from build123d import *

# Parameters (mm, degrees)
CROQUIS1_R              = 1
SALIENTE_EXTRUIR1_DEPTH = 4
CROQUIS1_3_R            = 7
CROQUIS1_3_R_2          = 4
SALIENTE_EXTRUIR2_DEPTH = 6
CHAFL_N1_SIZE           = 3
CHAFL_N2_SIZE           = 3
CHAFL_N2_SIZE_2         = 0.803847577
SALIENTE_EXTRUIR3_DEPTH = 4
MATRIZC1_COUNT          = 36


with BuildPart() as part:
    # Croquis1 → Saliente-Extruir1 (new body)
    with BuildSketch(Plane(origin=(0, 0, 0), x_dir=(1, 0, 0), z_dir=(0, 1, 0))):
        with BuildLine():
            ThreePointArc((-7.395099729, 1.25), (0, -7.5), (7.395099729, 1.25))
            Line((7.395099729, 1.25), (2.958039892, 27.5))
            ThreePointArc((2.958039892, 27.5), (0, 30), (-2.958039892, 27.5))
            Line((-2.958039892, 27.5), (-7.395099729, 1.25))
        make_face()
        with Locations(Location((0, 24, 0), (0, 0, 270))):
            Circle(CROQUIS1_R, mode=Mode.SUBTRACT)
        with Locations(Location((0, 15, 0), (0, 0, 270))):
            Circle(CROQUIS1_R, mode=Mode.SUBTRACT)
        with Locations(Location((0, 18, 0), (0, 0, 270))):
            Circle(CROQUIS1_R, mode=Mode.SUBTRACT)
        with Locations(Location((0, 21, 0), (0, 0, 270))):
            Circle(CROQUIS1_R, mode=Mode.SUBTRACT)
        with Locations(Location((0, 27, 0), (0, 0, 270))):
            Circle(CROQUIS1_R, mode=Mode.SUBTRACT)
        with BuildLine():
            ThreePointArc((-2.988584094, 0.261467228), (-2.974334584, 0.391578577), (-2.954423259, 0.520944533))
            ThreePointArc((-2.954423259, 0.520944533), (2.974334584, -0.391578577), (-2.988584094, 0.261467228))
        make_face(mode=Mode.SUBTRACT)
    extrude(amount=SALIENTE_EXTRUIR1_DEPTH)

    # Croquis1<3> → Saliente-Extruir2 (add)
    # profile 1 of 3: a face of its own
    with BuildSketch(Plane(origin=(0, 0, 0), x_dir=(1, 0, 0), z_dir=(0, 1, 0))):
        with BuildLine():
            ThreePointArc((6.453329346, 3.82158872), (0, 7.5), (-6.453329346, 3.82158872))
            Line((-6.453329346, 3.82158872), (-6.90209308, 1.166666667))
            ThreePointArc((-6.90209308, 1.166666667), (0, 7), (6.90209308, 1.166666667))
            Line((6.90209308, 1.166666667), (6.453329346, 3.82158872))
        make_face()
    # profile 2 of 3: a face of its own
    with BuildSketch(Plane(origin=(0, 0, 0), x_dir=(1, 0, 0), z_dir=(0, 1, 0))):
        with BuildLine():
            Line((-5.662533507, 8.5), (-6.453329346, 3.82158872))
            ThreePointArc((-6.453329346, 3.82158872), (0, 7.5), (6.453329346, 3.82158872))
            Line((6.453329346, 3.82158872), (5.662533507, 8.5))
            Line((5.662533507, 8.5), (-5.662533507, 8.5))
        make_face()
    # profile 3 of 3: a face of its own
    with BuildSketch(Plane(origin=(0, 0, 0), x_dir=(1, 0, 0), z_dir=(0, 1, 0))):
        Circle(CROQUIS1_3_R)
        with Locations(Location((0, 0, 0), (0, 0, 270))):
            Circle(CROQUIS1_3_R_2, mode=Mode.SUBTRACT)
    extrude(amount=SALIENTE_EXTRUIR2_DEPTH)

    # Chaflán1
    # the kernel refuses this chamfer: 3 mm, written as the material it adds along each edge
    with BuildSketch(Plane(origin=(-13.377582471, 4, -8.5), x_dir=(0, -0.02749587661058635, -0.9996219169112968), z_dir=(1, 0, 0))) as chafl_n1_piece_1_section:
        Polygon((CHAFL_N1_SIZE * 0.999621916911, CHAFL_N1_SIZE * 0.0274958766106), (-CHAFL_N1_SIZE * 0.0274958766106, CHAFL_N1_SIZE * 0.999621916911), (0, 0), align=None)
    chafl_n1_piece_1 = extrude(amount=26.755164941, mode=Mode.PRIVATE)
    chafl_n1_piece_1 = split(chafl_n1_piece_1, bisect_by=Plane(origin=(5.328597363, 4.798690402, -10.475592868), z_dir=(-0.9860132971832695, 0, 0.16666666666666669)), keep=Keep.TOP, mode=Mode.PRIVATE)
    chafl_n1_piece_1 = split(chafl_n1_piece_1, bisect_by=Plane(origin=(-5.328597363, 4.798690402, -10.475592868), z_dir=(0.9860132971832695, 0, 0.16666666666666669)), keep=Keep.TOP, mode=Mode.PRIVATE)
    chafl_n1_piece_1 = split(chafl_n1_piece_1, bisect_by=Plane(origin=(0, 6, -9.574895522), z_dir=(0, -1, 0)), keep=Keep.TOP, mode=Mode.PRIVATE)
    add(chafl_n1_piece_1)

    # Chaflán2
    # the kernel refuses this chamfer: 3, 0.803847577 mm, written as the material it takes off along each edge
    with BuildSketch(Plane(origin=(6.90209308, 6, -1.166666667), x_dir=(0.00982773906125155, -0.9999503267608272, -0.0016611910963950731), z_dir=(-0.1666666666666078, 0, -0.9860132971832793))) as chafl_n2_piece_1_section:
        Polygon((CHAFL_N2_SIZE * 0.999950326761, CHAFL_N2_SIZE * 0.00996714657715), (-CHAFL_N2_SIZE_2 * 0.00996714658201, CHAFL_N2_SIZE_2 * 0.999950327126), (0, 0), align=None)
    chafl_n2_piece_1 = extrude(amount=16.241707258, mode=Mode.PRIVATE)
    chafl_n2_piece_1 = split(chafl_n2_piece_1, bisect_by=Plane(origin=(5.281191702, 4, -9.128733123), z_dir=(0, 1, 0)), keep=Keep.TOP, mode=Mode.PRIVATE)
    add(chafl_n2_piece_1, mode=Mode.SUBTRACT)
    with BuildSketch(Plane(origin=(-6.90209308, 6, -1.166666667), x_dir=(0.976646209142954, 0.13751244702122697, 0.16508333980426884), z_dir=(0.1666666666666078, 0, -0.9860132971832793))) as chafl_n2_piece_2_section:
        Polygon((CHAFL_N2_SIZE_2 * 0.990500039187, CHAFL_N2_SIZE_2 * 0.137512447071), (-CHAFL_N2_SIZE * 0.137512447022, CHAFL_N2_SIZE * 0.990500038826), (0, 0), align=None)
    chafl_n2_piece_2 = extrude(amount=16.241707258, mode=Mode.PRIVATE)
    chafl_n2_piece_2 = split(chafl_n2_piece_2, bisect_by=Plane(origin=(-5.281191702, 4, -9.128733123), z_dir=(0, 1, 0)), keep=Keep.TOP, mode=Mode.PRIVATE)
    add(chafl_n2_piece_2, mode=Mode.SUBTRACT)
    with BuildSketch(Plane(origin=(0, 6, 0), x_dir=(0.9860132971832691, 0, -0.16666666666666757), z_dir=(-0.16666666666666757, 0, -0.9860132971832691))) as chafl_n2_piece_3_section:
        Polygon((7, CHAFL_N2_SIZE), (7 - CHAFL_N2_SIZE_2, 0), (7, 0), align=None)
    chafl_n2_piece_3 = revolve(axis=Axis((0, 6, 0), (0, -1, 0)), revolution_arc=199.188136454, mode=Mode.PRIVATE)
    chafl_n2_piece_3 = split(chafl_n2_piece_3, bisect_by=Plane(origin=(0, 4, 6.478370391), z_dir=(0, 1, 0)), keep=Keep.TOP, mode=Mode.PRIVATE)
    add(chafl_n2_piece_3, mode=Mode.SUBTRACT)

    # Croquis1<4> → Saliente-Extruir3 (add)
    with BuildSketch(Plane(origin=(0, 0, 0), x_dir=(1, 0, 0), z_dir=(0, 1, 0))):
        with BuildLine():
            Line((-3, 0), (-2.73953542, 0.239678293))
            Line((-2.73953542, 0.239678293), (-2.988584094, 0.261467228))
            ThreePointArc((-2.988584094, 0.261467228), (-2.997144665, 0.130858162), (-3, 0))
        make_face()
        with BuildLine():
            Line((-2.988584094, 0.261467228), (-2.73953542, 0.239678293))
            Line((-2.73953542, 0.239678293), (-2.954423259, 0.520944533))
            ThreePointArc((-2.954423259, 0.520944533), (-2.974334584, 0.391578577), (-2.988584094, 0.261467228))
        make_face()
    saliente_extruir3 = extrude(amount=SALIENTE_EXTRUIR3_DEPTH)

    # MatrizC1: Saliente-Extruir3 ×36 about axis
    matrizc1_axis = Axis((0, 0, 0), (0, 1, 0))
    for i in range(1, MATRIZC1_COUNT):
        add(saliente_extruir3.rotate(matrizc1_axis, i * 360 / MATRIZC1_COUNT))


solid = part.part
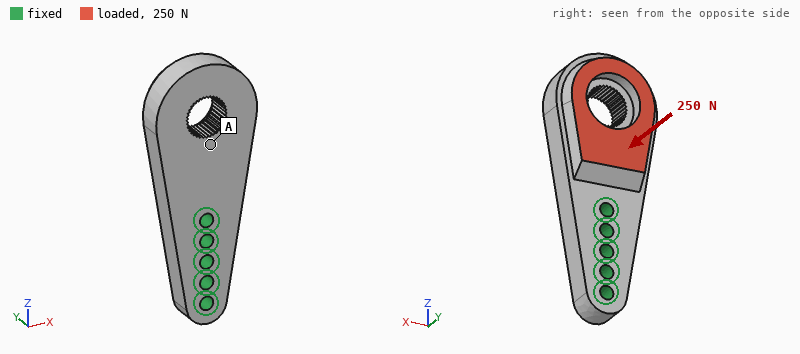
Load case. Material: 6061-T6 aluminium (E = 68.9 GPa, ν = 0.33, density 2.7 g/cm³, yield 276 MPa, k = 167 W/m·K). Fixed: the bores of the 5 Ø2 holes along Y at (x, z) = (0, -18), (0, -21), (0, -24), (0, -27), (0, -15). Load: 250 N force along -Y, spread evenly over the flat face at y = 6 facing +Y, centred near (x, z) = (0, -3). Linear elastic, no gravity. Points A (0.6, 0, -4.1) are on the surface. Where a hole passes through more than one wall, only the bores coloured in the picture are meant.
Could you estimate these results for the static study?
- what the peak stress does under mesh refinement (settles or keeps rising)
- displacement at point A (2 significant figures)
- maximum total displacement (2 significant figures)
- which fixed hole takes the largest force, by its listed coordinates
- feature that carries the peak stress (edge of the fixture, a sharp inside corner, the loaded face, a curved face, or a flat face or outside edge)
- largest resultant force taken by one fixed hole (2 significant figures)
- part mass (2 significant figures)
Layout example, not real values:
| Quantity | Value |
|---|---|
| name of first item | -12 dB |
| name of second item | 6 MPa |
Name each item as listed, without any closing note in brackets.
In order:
| Quantity | Value |
|---|---|
| what the peak stress does under mesh refinement | keeps rising |
| displacement at point A | 35 µm |
| maximum total displacement | 83 µm |
| which fixed hole takes the largest force, by its listed coordinates | (0, -15) |
| feature that carries the peak stress | edge of the fixture |
| largest resultant force taken by one fixed hole | 440 N |
| part mass | 4.5 g |
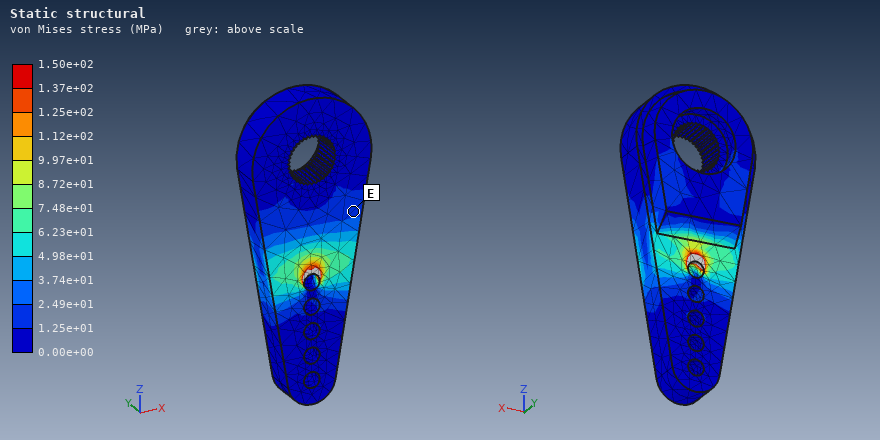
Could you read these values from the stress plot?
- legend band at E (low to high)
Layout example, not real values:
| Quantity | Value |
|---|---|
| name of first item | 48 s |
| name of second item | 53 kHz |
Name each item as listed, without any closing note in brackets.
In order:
| Quantity | Value |
|---|---|
| legend band at E | 1.25e+01 to 2.49e+01 MPa |
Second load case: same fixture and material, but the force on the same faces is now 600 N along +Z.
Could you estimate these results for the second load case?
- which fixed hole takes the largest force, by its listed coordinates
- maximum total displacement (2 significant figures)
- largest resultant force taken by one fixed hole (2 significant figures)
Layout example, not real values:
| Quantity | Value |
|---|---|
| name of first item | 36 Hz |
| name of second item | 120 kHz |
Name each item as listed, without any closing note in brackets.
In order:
| Quantity | Value |
|---|---|
| which fixed hole takes the largest force, by its listed coordinates | (0, -15) |
| maximum total displacement | 82 µm |
| largest resultant force taken by one fixed hole | 460 N |
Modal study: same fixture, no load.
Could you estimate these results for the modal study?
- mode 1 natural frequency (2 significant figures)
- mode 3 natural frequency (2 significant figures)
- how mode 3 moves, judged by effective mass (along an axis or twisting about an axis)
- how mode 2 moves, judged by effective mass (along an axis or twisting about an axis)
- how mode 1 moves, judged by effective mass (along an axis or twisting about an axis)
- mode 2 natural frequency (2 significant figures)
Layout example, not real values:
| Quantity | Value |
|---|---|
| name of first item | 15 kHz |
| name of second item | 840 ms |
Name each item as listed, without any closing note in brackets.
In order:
| Quantity | Value |
|---|---|
| mode 1 natural frequency | 6200 Hz |
| mode 3 natural frequency | 17 kHz |
| how mode 3 moves, judged by effective mass | twisting about Z |
| how mode 2 moves, judged by effective mass | along X |
| how mode 1 moves, judged by effective mass | along Y |
| mode 2 natural frequency | 10 kHz |
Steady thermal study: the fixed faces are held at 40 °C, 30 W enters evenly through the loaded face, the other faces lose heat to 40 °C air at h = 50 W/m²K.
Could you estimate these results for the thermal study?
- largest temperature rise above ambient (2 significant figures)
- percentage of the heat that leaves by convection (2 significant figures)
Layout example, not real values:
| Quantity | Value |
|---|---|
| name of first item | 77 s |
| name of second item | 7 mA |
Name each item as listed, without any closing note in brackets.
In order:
| Quantity | Value |
|---|---|
| largest temperature rise above ambient | 47 K |
| percentage of the heat that leaves by convection | 4.6 % |
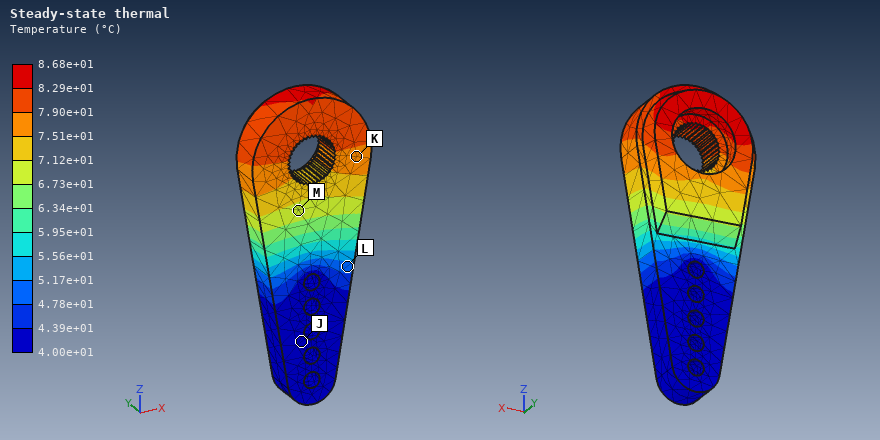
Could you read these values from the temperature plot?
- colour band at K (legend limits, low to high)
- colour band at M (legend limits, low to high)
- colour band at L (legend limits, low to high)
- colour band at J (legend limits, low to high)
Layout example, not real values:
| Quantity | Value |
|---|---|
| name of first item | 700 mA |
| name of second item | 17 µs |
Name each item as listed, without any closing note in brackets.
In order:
| Quantity | Value |
|---|---|
| colour band at K | 7.51e+01 to 7.90e+01 °C |
| colour band at M | 6.73e+01 to 7.12e+01 °C |
| colour band at L | 4.78e+01 to 5.17e+01 °C |
| colour band at J | 4.00e+01 to 4.39e+01 °C |
